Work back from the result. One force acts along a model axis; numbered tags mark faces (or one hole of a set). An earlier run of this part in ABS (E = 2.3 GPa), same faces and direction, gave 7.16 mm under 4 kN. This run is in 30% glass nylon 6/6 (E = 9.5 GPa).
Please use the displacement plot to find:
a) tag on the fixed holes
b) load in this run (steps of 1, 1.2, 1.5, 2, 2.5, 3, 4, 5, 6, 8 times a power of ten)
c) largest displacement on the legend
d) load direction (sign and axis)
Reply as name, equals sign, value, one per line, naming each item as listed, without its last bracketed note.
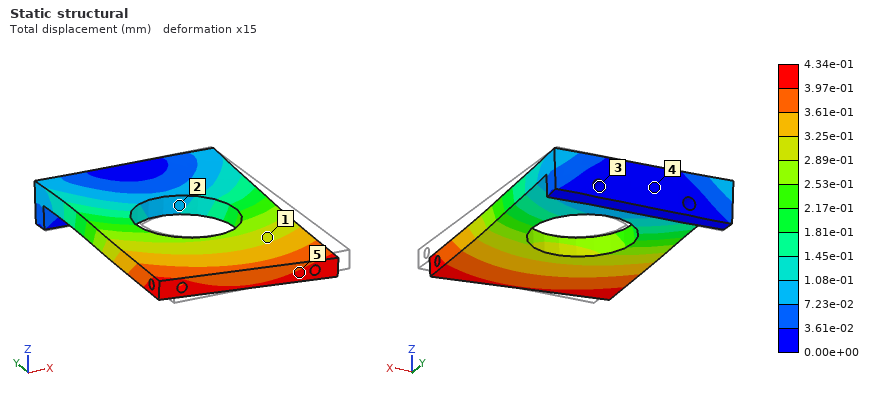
tag on the fixed holes = 3
load in this run = 1 kN
largest displacement on the legend = 4.34e-01 mm
load direction = -X
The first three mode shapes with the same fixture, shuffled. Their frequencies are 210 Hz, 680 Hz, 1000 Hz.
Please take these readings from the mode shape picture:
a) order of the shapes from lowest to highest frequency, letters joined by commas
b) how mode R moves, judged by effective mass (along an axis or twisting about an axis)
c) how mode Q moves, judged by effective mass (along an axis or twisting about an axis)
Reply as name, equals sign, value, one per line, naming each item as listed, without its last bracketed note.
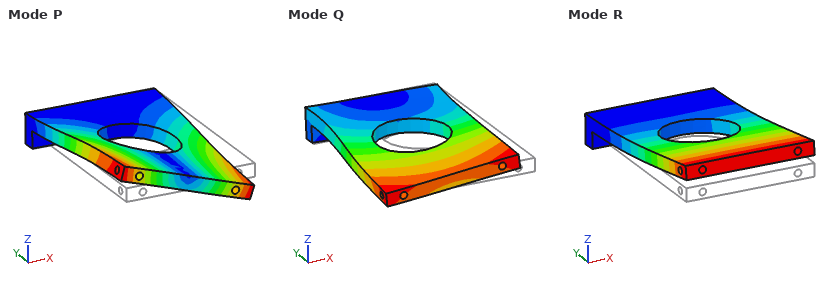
order of the shapes from lowest to highest frequency, letters joined by commas = R, P, Q
how mode R moves, judged by effective mass = along Z
how mode Q moves, judged by effective mass = along X
